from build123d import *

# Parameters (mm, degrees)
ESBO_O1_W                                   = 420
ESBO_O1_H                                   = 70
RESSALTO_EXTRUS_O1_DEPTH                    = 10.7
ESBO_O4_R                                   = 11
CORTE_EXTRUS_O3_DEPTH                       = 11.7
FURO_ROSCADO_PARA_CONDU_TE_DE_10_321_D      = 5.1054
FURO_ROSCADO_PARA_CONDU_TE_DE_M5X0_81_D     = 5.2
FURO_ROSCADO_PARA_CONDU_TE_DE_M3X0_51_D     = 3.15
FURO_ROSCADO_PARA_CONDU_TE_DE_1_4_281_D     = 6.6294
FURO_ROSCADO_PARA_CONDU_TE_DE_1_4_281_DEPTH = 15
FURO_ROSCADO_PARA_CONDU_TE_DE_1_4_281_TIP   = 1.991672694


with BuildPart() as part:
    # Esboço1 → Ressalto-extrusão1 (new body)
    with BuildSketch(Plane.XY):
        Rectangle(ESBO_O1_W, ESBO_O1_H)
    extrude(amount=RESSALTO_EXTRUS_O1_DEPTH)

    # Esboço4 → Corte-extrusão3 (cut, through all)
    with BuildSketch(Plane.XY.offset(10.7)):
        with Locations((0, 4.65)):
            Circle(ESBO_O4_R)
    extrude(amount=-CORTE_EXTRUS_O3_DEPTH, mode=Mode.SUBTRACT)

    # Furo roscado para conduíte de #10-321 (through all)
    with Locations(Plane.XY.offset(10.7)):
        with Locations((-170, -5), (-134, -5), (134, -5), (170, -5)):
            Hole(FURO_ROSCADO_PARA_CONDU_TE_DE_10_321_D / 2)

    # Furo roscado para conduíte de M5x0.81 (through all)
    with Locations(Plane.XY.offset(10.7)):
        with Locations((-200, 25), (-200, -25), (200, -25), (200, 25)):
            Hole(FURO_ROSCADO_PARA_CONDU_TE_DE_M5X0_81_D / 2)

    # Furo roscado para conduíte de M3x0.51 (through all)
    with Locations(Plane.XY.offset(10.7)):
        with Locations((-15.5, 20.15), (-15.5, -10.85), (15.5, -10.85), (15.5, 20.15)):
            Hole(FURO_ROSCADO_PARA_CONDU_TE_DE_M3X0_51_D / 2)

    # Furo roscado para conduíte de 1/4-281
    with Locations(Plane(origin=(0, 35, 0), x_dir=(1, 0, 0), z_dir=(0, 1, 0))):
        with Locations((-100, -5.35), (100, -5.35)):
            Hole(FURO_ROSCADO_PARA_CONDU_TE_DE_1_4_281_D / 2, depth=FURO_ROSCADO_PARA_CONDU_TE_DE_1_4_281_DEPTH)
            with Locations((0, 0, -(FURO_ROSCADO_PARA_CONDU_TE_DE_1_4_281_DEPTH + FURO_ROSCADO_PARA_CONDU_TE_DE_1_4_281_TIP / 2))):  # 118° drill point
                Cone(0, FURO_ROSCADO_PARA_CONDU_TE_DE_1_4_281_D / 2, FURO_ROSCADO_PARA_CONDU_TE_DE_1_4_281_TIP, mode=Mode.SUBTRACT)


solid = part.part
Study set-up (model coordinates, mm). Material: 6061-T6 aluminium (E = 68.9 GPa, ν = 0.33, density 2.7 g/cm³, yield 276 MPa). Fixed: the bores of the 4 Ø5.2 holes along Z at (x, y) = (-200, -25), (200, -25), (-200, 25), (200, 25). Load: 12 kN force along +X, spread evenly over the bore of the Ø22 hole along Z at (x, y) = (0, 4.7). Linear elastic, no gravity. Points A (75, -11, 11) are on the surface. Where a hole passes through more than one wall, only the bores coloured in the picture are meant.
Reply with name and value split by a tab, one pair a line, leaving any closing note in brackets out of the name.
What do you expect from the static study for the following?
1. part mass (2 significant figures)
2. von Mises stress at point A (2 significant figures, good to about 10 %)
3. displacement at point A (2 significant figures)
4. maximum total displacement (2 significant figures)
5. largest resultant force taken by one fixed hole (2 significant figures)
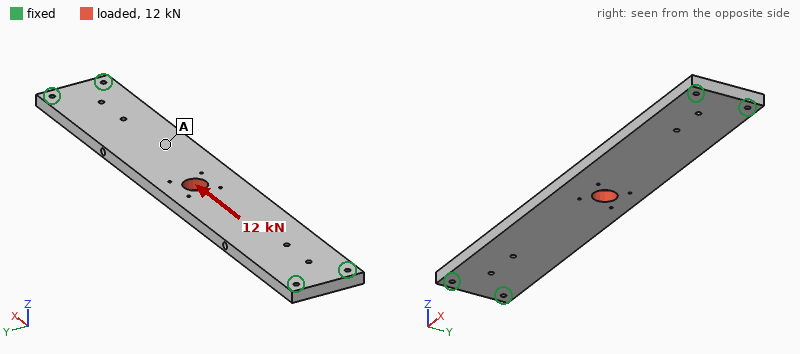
part mass	830 g
von Mises stress at point A	7.7 MPa
displacement at point A	17 µm
maximum total displacement	29 µm
largest resultant force taken by one fixed hole	3.3 kN
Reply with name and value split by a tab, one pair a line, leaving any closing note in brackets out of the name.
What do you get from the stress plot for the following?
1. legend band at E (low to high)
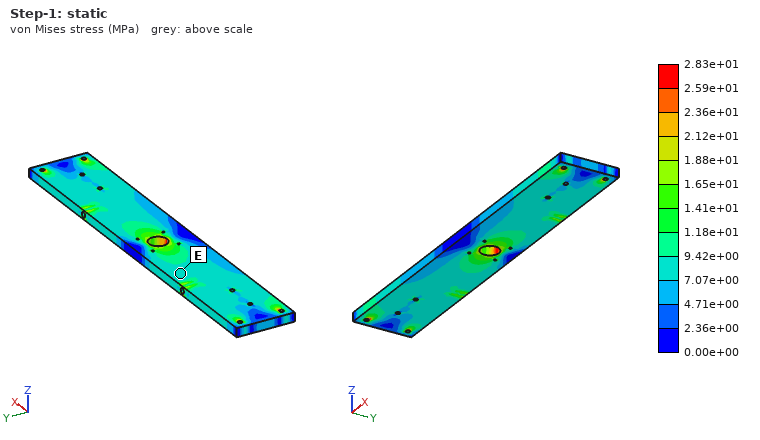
legend band at E	7.07e+00 to 9.42e+00 MPa
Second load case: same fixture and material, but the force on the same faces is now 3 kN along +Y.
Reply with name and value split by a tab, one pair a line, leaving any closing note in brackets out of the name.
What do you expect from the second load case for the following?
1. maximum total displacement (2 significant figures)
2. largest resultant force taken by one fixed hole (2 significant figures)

maximum total displacement	69 µm
largest resultant force taken by one fixed hole	3.0 kN
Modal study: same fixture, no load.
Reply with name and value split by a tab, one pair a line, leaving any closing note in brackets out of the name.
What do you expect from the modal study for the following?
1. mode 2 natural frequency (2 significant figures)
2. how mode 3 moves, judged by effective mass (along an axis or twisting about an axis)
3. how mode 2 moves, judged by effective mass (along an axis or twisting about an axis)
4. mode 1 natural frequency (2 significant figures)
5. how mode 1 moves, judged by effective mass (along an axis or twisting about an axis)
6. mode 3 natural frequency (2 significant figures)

mode 2 natural frequency	910 Hz
how mode 3 moves, judged by effective mass	twisting about X
how mode 2 moves, judged by effective mass	twisting about Y
mode 1 natural frequency	330 Hz
how mode 1 moves, judged by effective mass	along Z
mode 3 natural frequency	1200 Hz
